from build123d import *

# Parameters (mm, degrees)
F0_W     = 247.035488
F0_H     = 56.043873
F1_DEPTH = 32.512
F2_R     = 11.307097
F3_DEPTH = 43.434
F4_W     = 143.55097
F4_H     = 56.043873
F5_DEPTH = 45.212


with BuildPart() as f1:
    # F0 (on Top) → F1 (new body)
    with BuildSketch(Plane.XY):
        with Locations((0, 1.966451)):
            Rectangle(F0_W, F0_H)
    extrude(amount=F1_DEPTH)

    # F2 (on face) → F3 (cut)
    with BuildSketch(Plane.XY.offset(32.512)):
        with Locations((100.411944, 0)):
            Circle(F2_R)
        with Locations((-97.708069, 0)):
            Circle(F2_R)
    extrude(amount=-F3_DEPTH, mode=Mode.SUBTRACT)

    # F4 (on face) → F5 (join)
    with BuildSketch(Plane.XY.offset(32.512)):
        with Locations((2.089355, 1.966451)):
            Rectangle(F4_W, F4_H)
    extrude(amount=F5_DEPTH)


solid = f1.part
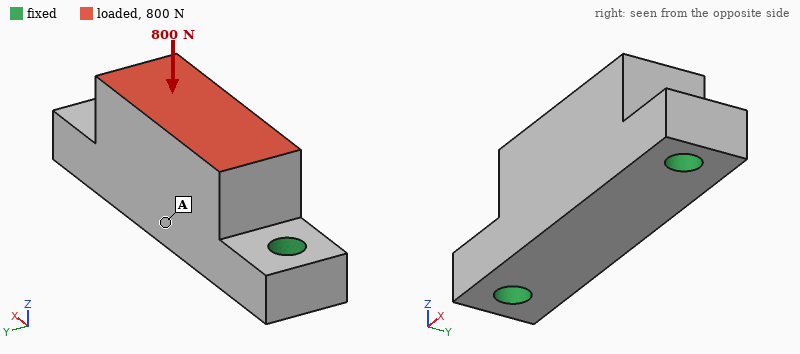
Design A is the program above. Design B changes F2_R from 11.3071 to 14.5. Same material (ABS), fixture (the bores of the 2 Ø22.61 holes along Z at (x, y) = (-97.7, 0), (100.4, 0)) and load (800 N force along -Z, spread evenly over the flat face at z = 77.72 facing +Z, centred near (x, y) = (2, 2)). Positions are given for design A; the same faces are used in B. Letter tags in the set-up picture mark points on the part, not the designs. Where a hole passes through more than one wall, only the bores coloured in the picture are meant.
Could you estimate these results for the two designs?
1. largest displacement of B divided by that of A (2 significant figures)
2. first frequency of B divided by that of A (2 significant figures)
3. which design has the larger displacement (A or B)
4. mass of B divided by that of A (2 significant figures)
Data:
0.86
1.1
A
0.98
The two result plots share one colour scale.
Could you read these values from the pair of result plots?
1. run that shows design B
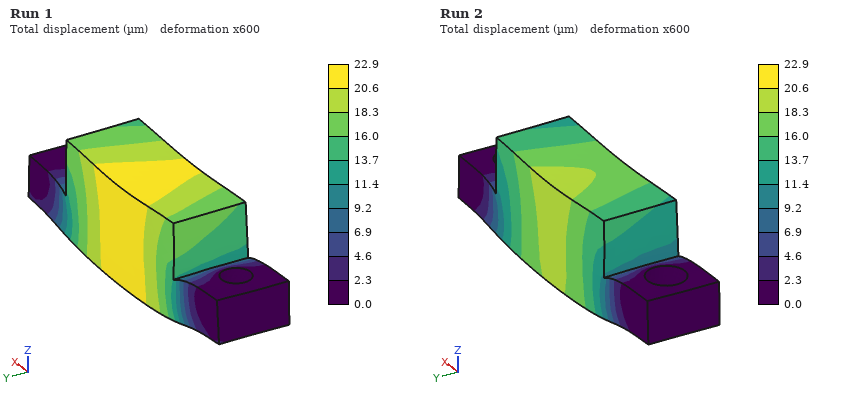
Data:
Run 2
